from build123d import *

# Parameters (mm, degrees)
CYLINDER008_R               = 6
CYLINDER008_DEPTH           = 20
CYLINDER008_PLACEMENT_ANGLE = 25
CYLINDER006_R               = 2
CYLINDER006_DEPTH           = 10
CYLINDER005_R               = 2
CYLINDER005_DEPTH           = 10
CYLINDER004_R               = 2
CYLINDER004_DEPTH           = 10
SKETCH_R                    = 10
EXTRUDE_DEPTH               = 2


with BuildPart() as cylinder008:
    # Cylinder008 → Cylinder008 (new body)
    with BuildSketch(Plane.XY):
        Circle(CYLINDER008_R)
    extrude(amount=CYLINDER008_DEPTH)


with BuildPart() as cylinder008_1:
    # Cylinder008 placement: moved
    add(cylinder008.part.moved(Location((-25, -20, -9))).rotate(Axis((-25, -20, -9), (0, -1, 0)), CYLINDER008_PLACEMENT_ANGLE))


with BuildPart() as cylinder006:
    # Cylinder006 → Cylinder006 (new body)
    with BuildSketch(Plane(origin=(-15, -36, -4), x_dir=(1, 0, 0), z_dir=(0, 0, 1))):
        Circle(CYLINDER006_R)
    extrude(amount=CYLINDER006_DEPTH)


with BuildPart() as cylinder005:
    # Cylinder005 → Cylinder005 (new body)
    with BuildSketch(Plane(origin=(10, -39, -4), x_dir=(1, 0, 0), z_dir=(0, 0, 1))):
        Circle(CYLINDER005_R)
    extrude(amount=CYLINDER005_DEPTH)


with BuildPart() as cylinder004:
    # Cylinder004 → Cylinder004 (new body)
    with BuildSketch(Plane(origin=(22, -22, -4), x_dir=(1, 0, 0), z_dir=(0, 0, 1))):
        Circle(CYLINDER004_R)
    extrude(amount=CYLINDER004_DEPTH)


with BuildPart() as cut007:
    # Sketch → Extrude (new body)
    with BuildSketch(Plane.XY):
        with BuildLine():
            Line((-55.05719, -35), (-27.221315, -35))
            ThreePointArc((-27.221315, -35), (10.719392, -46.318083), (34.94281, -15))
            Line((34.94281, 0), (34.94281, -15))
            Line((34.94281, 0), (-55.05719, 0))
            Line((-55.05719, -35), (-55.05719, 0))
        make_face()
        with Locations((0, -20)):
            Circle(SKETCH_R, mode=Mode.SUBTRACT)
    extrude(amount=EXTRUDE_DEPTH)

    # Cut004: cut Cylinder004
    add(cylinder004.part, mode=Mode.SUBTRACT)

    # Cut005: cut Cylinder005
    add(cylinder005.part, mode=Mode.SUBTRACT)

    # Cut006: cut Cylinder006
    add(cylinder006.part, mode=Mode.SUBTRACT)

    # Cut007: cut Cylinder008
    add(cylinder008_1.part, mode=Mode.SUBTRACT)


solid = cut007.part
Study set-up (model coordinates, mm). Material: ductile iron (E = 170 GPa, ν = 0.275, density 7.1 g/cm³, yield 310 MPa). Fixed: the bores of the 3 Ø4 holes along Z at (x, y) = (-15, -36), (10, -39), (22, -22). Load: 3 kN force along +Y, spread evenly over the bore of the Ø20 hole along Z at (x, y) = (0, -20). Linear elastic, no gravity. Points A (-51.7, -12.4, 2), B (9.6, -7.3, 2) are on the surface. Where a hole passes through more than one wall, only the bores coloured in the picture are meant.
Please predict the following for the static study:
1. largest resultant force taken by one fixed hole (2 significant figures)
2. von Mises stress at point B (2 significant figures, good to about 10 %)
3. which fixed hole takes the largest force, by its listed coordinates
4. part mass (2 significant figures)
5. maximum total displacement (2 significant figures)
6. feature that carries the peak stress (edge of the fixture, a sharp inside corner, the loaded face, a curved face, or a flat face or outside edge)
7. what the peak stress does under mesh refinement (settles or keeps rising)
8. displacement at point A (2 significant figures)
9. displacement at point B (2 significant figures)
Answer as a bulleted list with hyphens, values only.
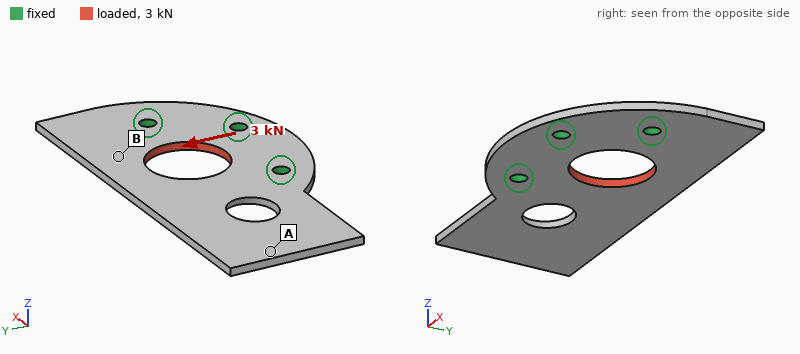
- 1.5 kN
- 28 MPa
- (-15, -36)
- 44 g
- 10 µm
- edge of the fixture
- keeps rising
- 4.5 µm
- 6.7 µm
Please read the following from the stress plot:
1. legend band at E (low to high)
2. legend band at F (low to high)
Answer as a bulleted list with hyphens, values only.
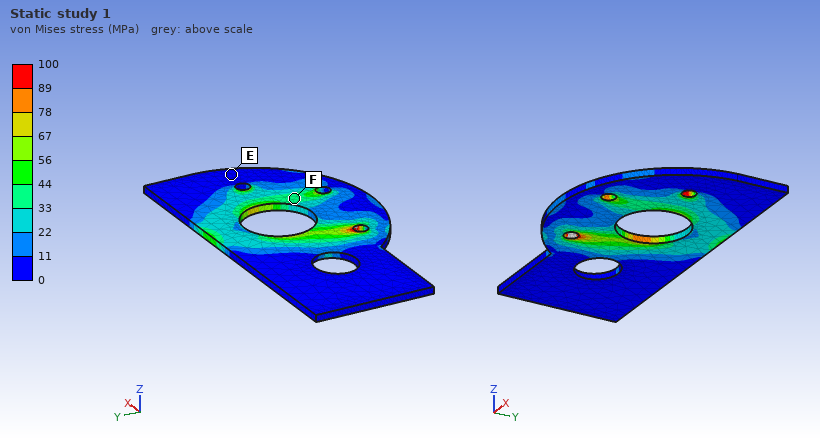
- 0 to 11 MPa
- 33 to 44 MPa
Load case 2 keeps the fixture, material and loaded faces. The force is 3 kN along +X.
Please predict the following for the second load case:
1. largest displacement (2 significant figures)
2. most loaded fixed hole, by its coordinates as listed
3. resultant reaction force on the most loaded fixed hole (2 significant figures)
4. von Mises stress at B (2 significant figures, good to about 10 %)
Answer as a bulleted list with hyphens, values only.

- 24 µm
- (22, -22)
- 1.8 kN
- 32 MPa
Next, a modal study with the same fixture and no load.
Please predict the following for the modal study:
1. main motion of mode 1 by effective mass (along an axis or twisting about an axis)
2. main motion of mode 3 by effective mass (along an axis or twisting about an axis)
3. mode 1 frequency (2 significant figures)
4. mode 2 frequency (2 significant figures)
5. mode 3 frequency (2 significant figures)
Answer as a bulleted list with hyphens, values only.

- along Z
- along Z
- 640 Hz
- 1500 Hz
- 2800 Hz
